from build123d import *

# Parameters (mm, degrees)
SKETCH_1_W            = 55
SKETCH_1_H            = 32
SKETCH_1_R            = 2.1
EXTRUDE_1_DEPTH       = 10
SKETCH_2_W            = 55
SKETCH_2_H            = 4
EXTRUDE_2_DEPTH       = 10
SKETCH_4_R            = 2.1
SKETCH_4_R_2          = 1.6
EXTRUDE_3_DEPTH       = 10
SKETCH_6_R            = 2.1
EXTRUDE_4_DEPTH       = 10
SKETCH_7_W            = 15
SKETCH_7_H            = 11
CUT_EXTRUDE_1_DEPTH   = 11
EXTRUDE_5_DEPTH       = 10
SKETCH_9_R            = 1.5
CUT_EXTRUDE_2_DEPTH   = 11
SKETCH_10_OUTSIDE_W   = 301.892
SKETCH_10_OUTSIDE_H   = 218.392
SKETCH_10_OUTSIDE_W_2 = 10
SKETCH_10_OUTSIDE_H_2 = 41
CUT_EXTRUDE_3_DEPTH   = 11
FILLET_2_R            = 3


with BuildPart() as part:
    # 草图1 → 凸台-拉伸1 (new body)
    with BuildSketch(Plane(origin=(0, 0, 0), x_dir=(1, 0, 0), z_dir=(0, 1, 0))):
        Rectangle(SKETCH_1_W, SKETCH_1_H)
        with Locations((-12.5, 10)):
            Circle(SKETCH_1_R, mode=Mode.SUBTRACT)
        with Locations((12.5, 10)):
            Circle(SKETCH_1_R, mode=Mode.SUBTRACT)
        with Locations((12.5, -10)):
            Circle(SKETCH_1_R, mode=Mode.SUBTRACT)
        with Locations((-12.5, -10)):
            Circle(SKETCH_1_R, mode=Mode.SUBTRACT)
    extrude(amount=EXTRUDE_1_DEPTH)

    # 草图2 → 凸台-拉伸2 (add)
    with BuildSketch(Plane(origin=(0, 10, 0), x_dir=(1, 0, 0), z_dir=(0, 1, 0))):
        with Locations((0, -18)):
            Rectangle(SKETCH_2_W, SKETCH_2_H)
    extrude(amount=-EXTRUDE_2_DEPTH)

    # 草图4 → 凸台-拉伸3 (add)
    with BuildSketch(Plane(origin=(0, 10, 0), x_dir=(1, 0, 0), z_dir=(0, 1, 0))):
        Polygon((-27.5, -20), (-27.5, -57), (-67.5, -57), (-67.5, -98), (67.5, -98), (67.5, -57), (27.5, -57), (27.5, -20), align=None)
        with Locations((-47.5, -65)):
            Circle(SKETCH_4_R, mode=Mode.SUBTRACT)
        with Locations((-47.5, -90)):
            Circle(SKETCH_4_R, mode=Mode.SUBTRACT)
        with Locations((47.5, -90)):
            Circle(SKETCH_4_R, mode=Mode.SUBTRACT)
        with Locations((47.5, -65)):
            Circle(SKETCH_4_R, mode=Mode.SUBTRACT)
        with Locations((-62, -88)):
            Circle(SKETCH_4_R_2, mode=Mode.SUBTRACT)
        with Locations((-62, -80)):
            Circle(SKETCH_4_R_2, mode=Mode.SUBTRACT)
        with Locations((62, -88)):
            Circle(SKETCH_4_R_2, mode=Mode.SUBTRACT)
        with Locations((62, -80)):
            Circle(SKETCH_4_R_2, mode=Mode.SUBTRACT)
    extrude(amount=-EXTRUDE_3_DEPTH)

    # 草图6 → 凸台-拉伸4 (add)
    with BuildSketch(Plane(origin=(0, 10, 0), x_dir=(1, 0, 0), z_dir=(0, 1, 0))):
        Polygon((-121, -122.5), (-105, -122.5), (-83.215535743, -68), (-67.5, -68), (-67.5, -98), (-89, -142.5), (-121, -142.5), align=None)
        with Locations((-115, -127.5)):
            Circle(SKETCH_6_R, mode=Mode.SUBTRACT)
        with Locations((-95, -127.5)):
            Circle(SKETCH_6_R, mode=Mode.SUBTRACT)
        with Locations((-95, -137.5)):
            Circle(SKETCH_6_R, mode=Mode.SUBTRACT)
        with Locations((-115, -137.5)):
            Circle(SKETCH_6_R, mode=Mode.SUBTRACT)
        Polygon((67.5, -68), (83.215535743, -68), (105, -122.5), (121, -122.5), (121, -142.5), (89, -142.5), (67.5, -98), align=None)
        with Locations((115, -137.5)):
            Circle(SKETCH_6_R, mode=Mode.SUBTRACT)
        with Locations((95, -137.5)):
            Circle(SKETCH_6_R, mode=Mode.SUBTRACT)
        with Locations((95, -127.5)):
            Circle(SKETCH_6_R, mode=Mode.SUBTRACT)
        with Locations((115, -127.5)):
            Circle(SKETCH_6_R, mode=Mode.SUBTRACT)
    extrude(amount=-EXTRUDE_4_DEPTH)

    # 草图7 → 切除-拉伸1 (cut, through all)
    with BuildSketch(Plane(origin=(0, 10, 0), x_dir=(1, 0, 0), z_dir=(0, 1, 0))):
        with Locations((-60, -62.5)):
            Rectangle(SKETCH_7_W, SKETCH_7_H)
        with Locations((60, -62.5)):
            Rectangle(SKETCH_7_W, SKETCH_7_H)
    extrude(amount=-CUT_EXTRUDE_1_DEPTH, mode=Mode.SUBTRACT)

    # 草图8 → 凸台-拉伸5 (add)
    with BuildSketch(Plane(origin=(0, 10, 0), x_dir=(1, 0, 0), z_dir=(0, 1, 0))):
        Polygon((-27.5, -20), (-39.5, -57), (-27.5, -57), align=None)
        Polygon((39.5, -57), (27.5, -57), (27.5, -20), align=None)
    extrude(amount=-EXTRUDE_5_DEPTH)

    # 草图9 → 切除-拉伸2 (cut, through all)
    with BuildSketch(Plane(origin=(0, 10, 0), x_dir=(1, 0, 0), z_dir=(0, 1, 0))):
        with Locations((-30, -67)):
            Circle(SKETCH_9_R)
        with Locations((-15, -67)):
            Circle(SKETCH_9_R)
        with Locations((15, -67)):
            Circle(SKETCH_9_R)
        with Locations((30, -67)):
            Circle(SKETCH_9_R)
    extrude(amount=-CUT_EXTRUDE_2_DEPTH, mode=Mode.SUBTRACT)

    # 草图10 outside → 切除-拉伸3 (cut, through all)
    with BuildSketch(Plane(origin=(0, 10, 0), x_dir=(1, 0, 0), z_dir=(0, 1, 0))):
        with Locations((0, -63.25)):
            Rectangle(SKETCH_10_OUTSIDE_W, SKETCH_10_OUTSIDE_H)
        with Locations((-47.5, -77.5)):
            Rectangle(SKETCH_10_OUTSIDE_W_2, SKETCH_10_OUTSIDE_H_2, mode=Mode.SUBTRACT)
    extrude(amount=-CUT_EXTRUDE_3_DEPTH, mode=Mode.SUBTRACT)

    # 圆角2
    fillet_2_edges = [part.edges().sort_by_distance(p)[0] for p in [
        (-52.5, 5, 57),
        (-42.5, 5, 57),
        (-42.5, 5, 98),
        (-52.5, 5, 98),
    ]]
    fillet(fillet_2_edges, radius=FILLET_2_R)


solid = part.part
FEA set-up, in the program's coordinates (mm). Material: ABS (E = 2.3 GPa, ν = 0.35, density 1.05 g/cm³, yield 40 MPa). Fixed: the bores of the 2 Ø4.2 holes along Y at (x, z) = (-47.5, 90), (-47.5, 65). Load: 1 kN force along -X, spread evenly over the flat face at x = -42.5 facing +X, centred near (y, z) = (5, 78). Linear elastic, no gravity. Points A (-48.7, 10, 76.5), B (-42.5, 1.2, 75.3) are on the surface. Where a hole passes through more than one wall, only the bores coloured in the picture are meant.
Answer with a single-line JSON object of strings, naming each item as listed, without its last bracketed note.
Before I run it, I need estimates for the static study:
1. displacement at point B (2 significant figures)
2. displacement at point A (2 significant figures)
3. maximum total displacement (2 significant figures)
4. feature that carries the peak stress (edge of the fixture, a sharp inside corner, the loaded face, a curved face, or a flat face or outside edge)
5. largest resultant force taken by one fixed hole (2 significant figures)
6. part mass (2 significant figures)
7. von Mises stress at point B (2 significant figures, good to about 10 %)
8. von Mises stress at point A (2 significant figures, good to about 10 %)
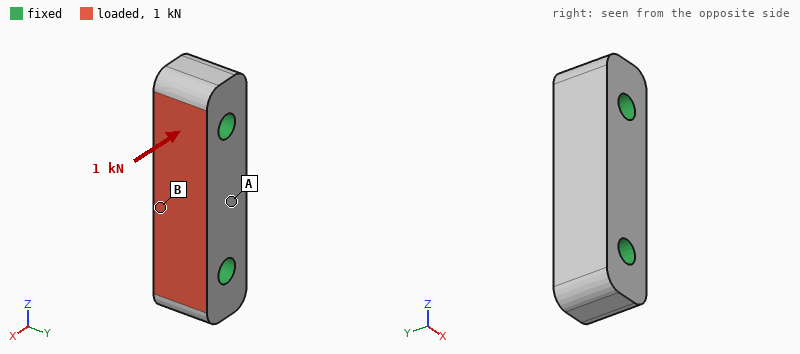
{"displacement at point B": "44 µm", "displacement at point A": "43 µm", "maximum total displacement": "47 µm", "feature that carries the peak stress": "edge of the fixture", "largest resultant force taken by one fixed hole": "500 N", "part mass": "3.9 g", "von Mises stress at point B": "5.5 MPa", "von Mises stress at point A": "1.6 MPa"}
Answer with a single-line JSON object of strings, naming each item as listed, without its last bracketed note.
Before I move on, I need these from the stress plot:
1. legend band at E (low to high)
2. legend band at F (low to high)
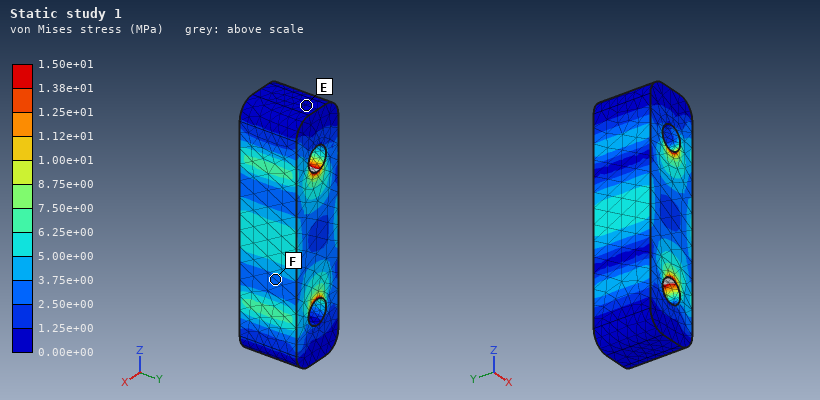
{"legend band at E": "0.00e+00 to 1.25e+00 MPa", "legend band at F": "2.50e+00 to 3.75e+00 MPa"}
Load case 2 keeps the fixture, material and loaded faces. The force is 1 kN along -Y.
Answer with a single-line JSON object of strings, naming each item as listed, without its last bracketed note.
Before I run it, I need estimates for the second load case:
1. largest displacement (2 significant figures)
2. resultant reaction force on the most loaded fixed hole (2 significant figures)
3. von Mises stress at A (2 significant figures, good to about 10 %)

{"largest displacement": "0.10 mm", "resultant reaction force on the most loaded fixed hole": "500 N", "von Mises stress at A": "4.6 MPa"}
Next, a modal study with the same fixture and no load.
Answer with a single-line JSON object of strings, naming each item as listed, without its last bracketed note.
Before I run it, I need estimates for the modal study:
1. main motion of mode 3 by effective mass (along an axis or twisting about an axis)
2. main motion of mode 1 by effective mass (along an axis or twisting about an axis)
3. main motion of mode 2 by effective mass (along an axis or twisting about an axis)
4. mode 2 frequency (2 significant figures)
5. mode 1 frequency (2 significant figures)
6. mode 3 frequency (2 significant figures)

{"main motion of mode 3 by effective mass": "twisting about Z", "main motion of mode 1 by effective mass": "along X", "main motion of mode 2 by effective mass": "along Y", "mode 2 frequency": "15 kHz", "mode 1 frequency": "14 kHz", "mode 3 frequency": "18 kHz"}
